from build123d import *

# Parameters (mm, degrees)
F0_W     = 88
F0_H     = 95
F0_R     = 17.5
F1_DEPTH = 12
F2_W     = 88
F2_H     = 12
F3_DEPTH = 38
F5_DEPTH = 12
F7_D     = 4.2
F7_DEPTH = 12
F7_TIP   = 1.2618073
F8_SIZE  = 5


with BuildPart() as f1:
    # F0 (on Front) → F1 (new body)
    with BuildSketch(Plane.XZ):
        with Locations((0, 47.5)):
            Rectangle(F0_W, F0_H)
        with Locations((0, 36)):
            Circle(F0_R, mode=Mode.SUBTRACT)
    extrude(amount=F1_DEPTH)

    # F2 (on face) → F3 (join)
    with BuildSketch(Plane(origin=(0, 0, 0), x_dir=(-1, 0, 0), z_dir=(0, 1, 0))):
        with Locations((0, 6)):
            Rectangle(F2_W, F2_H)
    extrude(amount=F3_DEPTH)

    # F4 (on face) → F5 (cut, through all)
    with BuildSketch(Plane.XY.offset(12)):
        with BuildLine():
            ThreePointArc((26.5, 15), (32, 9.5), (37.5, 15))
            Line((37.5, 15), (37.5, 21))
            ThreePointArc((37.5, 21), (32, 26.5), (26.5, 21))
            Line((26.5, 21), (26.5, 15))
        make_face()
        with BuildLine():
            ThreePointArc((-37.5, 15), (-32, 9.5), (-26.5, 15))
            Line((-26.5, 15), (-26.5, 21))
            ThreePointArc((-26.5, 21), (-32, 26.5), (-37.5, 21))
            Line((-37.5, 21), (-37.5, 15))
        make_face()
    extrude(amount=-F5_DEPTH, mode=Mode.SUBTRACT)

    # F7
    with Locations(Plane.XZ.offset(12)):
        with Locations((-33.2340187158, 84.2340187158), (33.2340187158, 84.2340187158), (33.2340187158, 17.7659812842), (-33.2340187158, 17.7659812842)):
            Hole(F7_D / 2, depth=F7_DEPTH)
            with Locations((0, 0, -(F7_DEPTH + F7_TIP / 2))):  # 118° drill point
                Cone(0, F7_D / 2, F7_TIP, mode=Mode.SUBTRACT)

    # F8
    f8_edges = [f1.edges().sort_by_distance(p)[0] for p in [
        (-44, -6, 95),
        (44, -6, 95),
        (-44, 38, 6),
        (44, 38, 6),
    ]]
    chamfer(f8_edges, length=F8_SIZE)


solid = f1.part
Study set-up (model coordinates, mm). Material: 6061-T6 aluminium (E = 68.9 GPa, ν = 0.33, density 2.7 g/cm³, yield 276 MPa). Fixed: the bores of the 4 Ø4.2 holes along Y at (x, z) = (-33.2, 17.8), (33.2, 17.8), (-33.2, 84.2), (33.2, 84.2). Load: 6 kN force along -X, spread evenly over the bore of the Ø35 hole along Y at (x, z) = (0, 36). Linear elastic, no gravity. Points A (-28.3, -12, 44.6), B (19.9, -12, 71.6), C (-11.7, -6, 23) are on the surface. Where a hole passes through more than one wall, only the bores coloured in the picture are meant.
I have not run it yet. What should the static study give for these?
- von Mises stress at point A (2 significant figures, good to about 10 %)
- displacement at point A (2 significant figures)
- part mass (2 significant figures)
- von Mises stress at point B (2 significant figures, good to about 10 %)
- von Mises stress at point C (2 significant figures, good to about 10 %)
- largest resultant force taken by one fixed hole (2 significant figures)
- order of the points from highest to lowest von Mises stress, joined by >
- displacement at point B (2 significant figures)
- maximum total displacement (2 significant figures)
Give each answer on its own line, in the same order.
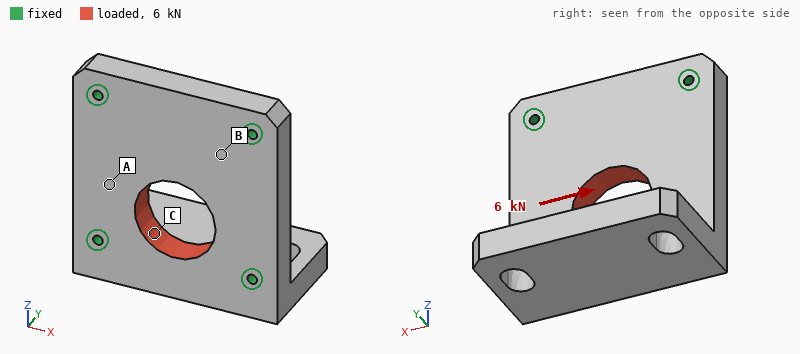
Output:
2.2 MPa
3.9 µm
330 g
4.7 MPa
7.8 MPa
1.9 kN
C > B > A
1.8 µm
4.5 µm
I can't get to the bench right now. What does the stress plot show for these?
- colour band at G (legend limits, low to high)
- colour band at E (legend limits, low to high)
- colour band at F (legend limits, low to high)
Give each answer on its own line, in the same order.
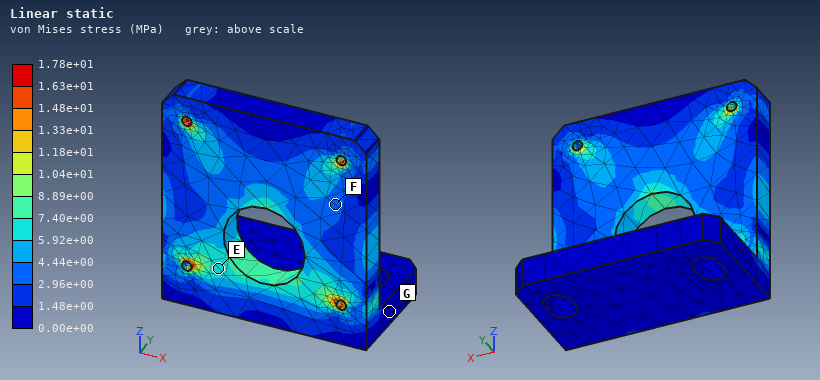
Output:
0.00e+00 to 1.48e+00 MPa
5.92e+00 to 7.40e+00 MPa
2.96e+00 to 4.44e+00 MPa
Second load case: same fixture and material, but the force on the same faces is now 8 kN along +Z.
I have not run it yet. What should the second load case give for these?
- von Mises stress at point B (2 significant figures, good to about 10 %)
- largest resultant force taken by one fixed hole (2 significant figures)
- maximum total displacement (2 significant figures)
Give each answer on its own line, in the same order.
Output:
5.6 MPa
2.4 kN
8.9 µm
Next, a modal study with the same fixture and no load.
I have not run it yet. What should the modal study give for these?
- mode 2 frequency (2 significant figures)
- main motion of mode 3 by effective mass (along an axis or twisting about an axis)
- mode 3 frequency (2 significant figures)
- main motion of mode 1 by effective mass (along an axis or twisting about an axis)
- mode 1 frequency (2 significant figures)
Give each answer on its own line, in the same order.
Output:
6000 Hz
along Y
8200 Hz
along Z
3100 Hz
